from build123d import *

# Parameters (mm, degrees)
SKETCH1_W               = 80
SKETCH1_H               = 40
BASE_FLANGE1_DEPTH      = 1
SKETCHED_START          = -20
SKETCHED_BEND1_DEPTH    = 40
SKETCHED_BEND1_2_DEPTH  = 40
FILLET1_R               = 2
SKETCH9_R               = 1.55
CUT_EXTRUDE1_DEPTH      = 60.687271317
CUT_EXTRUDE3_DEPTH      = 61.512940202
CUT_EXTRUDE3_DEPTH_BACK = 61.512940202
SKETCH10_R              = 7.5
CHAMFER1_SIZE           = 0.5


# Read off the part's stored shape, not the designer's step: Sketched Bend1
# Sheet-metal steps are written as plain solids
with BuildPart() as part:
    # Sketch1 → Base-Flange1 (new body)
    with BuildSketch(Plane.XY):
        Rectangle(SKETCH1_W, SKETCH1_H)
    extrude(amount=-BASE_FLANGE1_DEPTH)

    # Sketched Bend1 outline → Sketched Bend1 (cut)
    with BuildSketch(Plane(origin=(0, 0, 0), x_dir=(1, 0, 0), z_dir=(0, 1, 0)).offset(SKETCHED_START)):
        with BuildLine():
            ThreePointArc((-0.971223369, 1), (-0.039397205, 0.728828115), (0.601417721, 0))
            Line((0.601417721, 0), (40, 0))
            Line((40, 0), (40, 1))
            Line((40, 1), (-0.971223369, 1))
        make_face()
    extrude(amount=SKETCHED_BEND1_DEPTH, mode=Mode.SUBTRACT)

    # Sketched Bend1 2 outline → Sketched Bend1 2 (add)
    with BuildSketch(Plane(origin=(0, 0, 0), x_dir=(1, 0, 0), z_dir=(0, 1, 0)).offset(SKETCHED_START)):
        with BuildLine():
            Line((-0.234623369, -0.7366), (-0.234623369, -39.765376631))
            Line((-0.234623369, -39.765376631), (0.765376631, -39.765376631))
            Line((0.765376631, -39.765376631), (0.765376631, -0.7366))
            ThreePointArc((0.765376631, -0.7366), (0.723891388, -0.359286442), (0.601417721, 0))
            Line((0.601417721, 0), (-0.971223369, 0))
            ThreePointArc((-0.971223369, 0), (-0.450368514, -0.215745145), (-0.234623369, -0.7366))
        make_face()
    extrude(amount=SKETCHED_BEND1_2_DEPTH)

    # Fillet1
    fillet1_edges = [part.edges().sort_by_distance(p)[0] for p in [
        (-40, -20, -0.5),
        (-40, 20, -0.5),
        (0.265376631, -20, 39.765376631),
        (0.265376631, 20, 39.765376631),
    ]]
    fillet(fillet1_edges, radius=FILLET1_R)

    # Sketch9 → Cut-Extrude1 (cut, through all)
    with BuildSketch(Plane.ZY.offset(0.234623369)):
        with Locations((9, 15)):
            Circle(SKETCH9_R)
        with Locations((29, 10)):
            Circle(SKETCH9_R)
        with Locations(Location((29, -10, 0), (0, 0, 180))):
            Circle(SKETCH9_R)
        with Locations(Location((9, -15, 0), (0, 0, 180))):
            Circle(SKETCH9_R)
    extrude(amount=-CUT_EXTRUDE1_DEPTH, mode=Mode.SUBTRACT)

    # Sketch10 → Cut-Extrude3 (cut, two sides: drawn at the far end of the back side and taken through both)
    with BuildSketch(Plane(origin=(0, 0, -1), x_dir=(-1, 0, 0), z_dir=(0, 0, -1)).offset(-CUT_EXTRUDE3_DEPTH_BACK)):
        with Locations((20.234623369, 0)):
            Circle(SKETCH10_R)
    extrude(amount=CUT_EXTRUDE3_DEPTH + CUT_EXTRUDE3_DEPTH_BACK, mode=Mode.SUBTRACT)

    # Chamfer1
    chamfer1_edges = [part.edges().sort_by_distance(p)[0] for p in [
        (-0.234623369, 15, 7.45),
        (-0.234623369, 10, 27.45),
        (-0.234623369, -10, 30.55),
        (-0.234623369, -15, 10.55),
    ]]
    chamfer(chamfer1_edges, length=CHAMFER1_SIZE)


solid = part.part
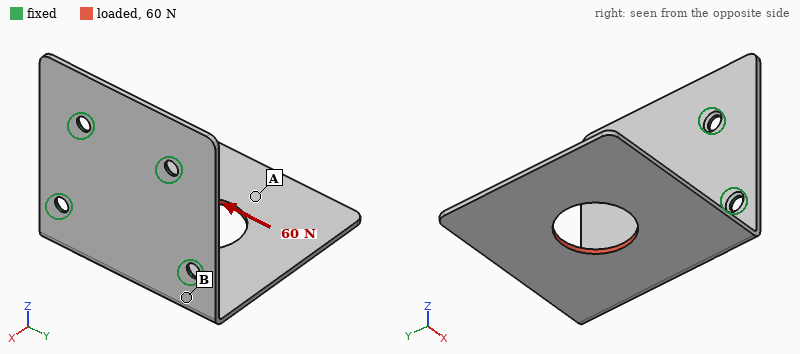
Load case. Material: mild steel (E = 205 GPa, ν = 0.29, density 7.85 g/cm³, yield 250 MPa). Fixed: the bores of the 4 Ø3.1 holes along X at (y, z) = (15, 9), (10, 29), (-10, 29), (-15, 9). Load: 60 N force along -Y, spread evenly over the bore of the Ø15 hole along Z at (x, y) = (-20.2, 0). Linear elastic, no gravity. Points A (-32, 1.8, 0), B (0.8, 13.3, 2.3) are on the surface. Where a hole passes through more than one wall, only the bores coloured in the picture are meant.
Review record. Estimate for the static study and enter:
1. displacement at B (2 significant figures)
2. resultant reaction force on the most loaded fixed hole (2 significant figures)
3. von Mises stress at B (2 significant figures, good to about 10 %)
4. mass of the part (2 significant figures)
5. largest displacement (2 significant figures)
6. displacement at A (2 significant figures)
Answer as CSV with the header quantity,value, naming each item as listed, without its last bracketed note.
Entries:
quantity,value
displacement at B,0.016 mm
resultant reaction force on the most loaded fixed hole,58 N
von Mises stress at B,41 MPa
mass of the part,23 g
largest displacement,0.10 mm
displacement at A,0.064 mm
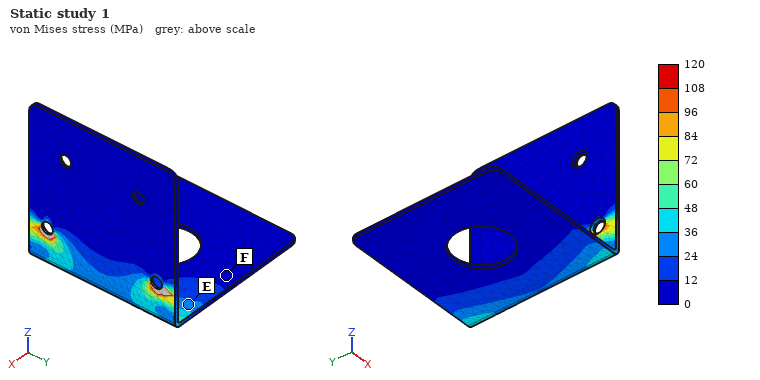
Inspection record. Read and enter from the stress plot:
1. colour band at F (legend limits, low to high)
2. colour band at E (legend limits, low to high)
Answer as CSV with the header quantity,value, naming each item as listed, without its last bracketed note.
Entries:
quantity,value
colour band at F,0 to 12 MPa
colour band at E,24 to 36 MPa
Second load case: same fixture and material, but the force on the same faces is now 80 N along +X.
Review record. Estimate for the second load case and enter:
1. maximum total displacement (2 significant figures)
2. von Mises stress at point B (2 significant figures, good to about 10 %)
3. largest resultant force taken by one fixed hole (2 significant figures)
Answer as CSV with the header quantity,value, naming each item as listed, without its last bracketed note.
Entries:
quantity,value
maximum total displacement,0.25 mm
von Mises stress at point B,35 MPa
largest resultant force taken by one fixed hole,56 N
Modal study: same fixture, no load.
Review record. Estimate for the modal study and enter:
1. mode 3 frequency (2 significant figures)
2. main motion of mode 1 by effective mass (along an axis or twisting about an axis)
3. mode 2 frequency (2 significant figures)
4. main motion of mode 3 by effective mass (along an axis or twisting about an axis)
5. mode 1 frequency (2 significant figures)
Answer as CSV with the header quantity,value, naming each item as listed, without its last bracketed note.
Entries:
quantity,value
mode 3 frequency,1600 Hz
main motion of mode 1 by effective mass,along Z
mode 2 frequency,1000 Hz
main motion of mode 3 by effective mass,along Y
mode 1 frequency,370 Hz
